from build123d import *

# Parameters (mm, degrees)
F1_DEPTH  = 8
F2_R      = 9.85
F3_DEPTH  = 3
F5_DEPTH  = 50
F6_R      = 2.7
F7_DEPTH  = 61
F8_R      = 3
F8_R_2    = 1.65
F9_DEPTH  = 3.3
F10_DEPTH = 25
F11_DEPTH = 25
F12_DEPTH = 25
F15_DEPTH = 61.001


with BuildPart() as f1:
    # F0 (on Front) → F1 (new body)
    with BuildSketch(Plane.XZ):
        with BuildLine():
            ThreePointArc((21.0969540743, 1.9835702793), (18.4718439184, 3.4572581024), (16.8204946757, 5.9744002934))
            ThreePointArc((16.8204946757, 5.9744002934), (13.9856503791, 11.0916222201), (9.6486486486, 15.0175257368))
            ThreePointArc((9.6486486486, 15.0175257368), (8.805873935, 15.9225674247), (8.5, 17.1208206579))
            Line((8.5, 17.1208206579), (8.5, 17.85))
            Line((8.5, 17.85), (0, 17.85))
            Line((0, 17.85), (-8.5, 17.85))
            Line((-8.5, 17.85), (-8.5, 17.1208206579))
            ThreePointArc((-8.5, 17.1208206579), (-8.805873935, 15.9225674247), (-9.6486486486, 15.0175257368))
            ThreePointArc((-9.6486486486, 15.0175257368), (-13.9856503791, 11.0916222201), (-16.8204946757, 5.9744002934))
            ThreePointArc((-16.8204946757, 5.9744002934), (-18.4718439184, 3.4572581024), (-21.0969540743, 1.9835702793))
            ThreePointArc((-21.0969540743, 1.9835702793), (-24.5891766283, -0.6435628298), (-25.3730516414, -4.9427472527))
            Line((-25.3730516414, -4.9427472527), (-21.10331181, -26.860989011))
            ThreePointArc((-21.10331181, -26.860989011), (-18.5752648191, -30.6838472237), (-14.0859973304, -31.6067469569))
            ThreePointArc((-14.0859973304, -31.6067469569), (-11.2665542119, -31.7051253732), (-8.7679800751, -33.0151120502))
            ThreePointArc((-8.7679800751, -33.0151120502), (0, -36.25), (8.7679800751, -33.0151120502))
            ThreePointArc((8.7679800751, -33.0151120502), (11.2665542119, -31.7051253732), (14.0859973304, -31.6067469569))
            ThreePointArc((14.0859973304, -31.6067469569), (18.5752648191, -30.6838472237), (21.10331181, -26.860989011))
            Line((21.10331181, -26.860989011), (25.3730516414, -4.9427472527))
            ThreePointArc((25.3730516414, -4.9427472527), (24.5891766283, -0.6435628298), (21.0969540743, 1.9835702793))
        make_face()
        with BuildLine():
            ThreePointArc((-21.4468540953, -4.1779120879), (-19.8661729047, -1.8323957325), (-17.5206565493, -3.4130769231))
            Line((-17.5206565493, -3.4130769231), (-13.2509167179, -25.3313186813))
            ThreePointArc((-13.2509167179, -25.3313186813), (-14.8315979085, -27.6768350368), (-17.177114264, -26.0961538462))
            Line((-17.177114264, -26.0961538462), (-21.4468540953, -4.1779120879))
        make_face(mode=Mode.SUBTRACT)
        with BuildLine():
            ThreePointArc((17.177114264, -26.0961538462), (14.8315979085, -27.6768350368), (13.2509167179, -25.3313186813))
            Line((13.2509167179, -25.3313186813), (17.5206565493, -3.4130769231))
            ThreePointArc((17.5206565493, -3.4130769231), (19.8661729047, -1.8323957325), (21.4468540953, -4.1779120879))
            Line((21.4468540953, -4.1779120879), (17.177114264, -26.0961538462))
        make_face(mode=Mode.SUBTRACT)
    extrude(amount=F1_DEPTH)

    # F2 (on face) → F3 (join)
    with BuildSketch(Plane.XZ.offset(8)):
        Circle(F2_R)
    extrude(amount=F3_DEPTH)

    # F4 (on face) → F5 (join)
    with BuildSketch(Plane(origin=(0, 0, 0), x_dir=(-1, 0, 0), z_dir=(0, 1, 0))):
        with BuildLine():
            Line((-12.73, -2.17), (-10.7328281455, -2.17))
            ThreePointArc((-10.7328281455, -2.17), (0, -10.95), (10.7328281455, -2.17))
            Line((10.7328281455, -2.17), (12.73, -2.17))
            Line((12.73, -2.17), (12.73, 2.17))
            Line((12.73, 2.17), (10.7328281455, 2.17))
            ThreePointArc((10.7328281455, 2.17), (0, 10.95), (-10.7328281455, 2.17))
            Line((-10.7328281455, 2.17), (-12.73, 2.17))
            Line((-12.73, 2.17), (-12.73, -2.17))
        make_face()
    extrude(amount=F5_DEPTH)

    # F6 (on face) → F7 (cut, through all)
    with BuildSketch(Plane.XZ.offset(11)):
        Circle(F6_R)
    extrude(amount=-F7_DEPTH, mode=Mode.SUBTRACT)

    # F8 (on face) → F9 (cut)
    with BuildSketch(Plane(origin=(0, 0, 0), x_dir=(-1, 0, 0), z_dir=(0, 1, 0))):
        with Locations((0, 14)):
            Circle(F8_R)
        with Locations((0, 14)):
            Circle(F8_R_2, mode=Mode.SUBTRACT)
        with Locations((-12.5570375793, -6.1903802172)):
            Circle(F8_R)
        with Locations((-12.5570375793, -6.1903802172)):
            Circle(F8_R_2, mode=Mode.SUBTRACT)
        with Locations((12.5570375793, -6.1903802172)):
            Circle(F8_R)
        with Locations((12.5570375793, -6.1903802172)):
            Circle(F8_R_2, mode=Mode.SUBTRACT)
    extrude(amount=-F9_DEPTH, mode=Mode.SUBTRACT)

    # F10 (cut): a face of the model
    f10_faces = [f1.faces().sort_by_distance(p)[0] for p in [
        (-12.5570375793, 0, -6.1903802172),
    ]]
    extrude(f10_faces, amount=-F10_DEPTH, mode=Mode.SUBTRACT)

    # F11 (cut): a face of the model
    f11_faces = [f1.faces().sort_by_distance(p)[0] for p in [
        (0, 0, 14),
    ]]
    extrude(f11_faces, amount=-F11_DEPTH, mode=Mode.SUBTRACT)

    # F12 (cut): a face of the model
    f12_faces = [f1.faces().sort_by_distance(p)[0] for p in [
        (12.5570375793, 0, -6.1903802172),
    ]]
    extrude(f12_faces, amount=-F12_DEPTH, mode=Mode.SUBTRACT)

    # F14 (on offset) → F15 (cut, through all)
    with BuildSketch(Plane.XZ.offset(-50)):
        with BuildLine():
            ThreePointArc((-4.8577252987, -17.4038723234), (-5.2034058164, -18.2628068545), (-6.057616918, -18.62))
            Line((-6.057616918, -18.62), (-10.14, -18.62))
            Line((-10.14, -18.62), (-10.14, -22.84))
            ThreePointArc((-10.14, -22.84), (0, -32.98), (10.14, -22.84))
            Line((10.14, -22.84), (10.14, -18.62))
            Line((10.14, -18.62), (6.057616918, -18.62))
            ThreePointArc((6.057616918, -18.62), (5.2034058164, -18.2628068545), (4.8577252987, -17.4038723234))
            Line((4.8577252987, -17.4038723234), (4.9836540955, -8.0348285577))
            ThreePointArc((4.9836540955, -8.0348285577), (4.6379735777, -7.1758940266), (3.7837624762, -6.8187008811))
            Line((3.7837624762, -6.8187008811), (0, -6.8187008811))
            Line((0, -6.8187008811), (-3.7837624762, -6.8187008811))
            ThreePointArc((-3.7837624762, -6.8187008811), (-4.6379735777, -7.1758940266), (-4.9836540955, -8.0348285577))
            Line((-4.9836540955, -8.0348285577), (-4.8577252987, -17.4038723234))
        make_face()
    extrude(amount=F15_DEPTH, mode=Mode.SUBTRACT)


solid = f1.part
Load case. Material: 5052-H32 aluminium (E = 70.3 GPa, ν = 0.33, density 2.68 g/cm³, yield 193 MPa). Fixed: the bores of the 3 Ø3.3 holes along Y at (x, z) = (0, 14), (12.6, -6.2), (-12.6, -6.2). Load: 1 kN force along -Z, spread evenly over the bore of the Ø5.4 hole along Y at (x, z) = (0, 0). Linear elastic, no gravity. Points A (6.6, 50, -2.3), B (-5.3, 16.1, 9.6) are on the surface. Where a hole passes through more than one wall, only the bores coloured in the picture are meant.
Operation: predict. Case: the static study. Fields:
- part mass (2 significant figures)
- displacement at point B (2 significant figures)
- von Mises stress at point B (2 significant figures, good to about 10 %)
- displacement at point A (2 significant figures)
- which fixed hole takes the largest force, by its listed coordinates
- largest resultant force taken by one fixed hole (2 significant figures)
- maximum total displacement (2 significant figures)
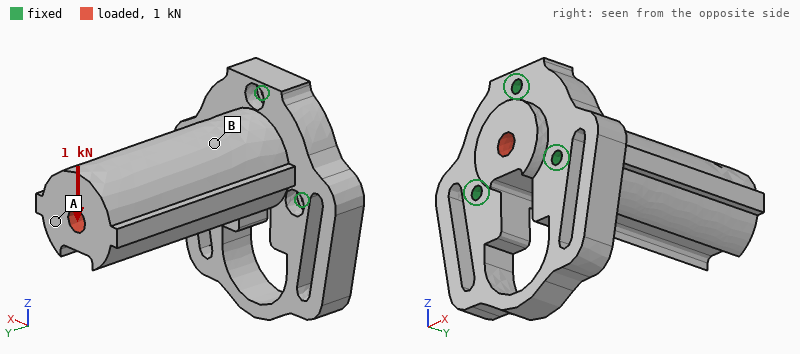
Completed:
77 g
16 µm
10 MPa
48 µm
(0, 14)
1.3 kN
49 µm
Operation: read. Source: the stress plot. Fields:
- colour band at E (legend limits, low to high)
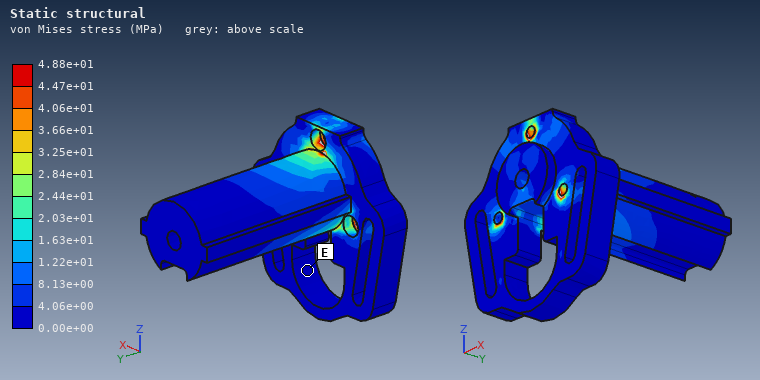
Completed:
0.00e+00 to 4.06e+00 MPa
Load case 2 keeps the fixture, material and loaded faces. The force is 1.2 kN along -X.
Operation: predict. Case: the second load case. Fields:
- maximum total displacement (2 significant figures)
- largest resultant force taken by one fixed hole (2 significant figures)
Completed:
44 µm
1.3 kN
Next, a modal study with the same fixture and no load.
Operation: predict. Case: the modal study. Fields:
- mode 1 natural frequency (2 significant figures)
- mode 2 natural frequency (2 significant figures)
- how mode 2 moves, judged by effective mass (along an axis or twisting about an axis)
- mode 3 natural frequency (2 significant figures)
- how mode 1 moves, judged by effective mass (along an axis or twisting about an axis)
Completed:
3800 Hz
4300 Hz
along X
6500 Hz
along Z
